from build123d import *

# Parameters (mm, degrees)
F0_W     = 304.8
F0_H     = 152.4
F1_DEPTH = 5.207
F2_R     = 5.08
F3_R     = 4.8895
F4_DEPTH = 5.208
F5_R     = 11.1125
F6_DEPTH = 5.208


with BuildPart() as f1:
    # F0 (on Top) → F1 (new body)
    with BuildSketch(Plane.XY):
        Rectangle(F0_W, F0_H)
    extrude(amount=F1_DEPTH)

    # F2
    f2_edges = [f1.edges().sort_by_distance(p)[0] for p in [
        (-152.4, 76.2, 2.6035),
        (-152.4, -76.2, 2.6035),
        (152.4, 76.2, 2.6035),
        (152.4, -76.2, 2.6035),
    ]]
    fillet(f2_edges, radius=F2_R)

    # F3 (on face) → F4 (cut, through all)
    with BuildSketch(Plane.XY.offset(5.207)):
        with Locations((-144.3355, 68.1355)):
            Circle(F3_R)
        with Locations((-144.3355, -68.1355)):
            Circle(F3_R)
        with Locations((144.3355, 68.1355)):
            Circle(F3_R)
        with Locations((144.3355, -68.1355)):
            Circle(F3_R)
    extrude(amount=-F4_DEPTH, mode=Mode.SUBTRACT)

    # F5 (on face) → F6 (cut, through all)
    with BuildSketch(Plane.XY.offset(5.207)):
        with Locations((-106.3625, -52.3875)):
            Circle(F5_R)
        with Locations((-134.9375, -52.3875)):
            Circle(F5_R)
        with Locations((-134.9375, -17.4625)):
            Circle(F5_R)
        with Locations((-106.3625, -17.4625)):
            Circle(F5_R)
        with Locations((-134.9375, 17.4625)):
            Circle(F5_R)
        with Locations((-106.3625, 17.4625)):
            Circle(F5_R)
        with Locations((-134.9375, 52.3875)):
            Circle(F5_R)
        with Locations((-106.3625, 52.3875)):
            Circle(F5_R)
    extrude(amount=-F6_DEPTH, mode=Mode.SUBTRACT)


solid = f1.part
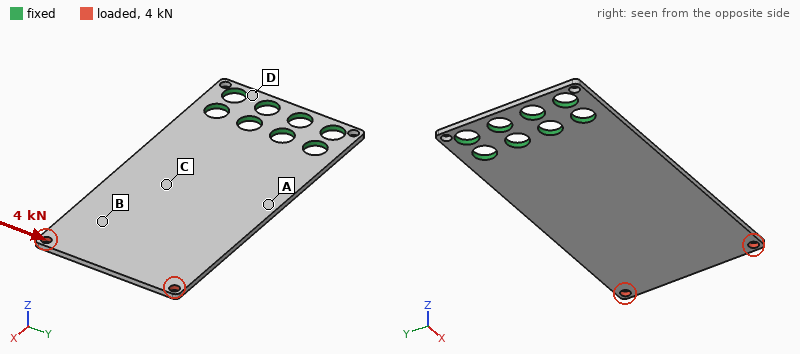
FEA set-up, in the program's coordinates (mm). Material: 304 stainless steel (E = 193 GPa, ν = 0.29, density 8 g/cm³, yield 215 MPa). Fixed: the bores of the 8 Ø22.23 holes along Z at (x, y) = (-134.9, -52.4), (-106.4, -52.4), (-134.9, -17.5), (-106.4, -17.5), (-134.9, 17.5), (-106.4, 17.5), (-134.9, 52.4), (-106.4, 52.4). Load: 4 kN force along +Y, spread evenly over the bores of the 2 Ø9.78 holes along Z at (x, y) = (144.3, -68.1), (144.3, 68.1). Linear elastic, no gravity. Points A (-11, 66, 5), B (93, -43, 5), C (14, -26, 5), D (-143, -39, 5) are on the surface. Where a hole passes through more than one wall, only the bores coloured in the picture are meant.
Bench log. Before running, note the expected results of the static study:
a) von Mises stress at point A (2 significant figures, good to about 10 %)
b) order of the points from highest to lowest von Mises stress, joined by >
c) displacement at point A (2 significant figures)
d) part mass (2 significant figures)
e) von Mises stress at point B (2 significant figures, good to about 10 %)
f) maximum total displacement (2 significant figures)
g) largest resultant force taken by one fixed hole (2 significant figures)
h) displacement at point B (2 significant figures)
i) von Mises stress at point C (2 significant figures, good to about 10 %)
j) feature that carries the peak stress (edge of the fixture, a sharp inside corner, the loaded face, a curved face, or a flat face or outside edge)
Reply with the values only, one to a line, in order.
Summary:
27 MPa
A > C > B > D
0.026 mm
1.8 kg
9.7 MPa
0.10 mm
7.4 kN
0.065 mm
15 MPa
edge of the fixture
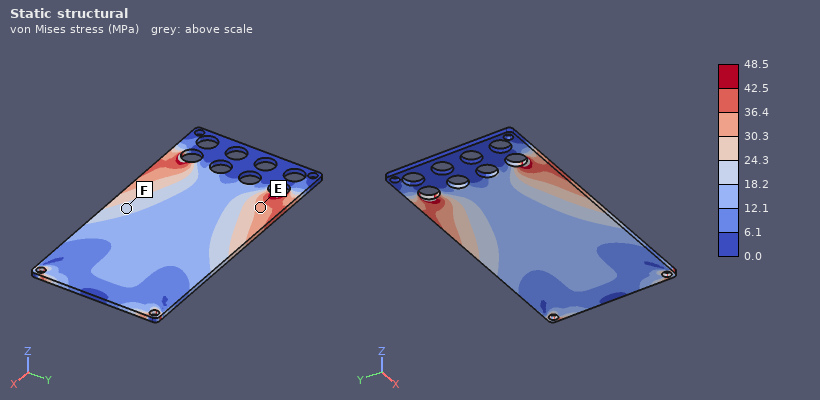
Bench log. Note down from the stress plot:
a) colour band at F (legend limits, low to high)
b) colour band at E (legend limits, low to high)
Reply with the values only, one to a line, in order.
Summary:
18.2 to 24.3 MPa
30.3 to 36.4 MPa
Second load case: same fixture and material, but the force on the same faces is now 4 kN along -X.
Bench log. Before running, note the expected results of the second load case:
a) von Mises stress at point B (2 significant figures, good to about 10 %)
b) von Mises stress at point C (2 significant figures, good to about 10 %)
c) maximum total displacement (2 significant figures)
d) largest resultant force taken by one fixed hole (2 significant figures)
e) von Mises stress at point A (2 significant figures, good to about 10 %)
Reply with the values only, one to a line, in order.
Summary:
6.2 MPa
4.8 MPa
13 µm
1.1 kN
4.9 MPa
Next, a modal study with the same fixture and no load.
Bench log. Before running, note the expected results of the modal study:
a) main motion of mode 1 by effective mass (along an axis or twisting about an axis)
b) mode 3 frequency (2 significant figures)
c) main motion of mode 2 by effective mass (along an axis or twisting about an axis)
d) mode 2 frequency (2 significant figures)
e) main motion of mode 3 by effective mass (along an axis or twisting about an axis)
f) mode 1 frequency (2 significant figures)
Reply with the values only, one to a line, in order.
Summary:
along Z
420 Hz
twisting about X
250 Hz
along Z
68 Hz
